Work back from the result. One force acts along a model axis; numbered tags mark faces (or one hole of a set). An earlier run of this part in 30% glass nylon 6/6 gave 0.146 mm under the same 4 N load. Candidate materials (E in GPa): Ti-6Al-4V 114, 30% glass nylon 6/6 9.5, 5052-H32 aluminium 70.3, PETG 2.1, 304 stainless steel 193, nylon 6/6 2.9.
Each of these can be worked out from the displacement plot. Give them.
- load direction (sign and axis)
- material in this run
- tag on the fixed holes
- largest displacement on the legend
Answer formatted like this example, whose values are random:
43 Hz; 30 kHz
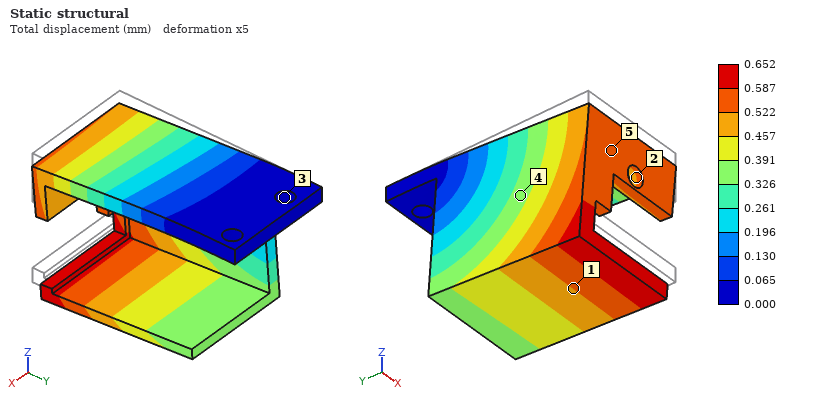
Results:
-Z; PETG; 3; 0.652 mm
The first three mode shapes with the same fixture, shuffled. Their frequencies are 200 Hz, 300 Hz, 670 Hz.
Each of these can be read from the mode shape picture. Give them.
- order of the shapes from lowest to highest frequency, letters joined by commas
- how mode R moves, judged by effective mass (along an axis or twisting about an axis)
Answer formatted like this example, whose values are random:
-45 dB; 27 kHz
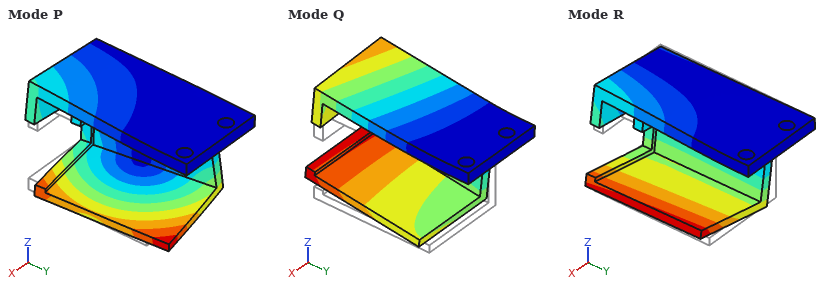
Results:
Q, R, P; along X
